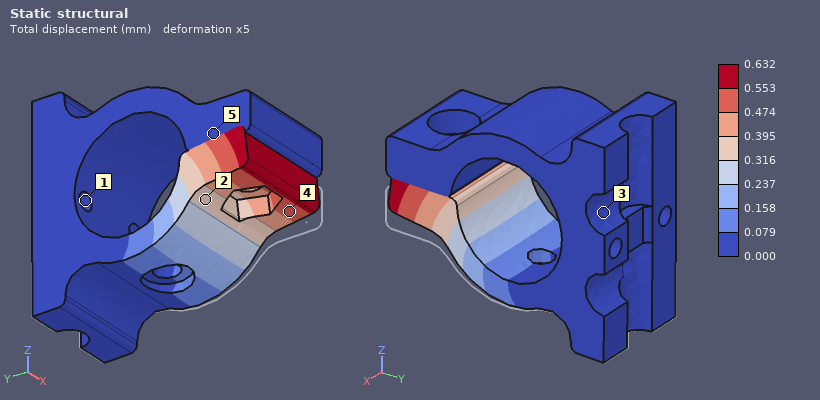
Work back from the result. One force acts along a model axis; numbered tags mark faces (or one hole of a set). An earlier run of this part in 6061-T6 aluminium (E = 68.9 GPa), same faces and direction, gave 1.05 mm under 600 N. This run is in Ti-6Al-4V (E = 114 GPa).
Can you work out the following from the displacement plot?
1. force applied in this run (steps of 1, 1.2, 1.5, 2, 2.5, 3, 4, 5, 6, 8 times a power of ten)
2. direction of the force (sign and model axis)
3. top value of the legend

600 N
+Z
0.632 mm
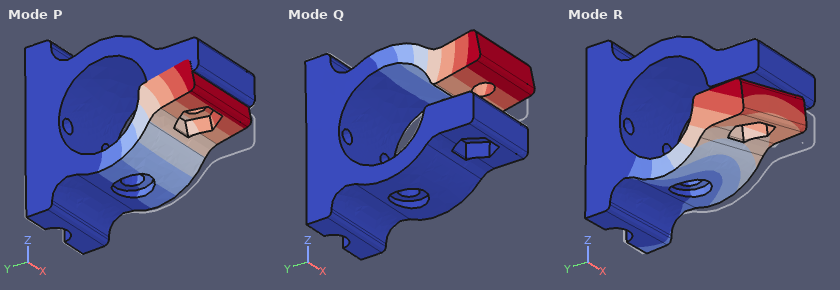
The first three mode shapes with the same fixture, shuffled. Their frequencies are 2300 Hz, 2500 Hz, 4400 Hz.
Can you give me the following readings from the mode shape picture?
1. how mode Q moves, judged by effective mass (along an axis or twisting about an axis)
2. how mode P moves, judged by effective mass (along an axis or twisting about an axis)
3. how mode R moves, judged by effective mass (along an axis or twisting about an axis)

along Z
along Z
along X
